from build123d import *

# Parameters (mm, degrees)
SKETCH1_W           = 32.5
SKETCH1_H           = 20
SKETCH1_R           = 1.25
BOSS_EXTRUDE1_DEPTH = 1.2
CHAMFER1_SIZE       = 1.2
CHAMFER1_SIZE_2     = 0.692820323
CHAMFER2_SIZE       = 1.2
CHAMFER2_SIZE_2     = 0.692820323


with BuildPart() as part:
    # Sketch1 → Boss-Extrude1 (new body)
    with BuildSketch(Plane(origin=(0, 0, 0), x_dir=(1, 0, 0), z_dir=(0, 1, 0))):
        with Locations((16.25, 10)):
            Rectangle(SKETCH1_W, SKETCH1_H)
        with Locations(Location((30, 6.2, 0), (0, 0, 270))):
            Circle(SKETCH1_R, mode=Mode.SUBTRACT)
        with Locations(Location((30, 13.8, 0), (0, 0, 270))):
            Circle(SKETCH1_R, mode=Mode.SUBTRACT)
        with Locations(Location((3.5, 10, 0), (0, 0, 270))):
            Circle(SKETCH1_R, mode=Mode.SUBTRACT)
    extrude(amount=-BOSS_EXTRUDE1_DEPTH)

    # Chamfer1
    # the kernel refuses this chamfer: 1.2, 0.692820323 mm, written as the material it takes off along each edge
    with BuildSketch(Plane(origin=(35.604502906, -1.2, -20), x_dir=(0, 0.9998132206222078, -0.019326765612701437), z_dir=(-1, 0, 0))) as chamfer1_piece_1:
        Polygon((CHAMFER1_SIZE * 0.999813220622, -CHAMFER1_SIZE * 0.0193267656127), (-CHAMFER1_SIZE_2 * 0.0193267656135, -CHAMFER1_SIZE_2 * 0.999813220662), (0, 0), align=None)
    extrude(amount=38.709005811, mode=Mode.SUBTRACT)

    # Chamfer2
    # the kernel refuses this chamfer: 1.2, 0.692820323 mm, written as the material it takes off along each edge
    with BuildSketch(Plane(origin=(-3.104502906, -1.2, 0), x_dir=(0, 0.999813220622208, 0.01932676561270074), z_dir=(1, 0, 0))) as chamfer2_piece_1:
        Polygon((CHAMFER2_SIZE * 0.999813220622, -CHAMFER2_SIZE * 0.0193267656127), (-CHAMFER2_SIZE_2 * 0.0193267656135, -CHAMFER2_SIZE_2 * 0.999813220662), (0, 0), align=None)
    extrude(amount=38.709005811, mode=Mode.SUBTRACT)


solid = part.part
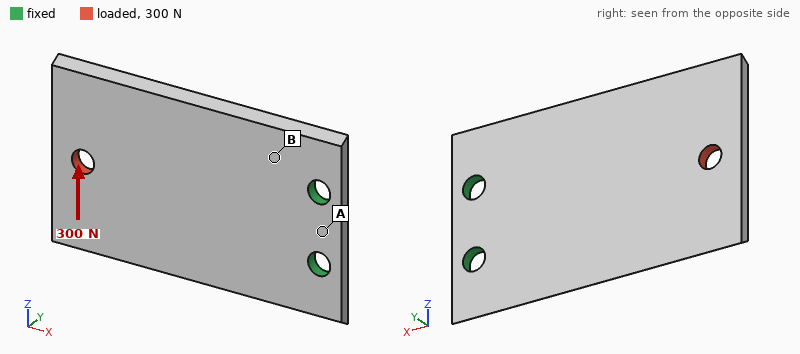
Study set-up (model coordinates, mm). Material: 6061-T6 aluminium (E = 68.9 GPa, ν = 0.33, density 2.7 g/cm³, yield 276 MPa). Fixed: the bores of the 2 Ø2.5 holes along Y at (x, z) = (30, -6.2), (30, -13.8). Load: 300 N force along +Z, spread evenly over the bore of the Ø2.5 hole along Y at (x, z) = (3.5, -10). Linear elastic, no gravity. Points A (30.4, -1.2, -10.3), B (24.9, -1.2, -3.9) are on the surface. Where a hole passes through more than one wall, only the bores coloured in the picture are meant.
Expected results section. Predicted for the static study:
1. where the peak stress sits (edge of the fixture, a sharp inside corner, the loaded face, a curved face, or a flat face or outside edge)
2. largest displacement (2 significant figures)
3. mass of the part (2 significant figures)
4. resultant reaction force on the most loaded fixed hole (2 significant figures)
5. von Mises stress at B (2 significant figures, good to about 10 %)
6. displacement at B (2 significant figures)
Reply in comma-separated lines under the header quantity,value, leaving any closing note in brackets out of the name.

quantity,value
where the peak stress sits,edge of the fixture
largest displacement,0.10 mm
mass of the part,2.0 g
resultant reaction force on the most loaded fixed hole,800 N
von Mises stress at B,68 MPa
displacement at B,0.016 mm
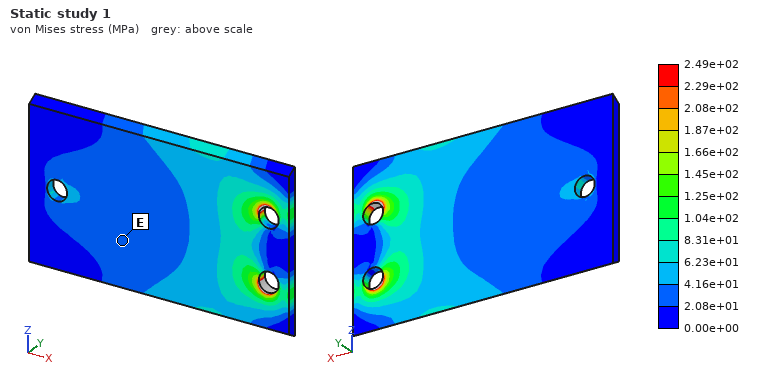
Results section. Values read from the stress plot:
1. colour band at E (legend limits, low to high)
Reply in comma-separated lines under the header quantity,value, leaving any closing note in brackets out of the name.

quantity,value
colour band at E,2.08e+01 to 4.16e+01 MPa
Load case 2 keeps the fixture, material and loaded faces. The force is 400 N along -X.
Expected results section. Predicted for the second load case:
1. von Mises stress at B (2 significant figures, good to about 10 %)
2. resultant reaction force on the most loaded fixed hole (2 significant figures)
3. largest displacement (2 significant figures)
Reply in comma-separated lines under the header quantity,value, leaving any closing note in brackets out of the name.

quantity,value
von Mises stress at B,19 MPa
resultant reaction force on the most loaded fixed hole,200 N
largest displacement,12 µm
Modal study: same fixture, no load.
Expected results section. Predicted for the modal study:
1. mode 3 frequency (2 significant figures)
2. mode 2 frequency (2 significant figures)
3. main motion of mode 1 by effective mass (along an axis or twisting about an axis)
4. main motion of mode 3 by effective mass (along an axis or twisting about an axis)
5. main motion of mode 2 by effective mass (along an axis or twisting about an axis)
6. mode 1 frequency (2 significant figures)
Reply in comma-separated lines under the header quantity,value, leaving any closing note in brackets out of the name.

quantity,value
mode 3 frequency,7000 Hz
mode 2 frequency,3700 Hz
main motion of mode 1 by effective mass,along Y
main motion of mode 3 by effective mass,along Y
main motion of mode 2 by effective mass,twisting about X
mode 1 frequency,1200 Hz
